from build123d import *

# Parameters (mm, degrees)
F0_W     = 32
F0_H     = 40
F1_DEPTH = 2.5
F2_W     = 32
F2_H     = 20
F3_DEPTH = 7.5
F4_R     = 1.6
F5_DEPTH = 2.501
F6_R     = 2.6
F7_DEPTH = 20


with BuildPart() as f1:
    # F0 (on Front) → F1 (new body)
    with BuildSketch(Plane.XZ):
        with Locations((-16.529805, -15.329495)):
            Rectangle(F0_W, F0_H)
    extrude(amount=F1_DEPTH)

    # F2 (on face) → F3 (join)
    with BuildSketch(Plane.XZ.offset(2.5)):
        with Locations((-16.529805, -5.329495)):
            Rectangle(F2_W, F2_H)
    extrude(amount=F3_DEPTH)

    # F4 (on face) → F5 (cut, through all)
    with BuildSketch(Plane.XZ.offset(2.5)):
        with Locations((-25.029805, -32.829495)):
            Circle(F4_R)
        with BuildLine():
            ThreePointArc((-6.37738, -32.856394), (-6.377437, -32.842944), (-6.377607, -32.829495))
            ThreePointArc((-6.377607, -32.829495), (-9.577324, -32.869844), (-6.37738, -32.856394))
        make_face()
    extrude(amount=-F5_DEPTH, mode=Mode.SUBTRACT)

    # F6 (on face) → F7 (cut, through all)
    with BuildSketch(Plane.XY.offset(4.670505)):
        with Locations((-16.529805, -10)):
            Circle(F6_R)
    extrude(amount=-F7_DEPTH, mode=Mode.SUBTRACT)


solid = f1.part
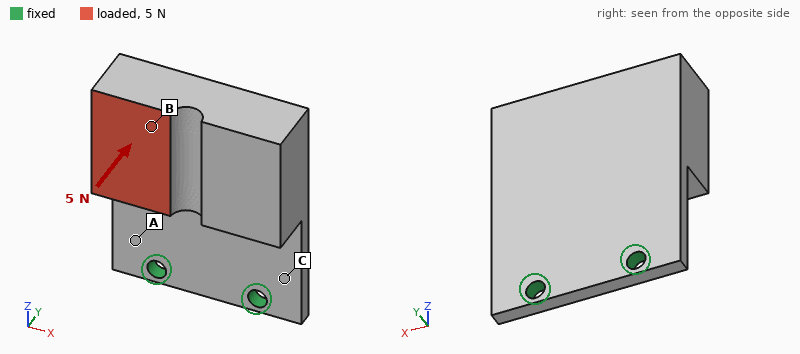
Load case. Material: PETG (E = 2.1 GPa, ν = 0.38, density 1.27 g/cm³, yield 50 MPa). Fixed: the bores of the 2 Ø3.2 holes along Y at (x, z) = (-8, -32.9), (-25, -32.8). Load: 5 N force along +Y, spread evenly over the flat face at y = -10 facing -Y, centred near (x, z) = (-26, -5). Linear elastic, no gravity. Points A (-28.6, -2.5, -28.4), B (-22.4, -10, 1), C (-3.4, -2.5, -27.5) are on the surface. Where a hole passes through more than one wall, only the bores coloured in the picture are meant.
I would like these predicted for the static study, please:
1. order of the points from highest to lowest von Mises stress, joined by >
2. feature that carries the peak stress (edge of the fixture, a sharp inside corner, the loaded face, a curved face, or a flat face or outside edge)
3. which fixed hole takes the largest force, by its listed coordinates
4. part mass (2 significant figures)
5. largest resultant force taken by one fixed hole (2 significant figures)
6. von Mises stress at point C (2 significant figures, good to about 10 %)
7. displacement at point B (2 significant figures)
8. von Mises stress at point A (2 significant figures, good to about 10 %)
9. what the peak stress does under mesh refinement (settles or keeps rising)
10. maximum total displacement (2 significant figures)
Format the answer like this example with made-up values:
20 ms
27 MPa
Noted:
A > C > B
edge of the fixture
(-25, -32.8)
9.8 g
4.8 N
2.7 MPa
0.52 mm
3.7 MPa
keeps rising
0.61 mm
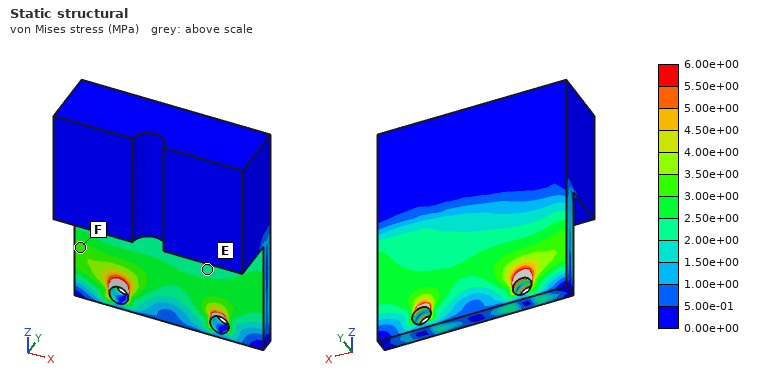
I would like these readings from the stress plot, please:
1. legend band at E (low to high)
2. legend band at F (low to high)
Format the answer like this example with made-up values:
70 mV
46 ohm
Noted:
2.00e+00 to 2.50e+00 MPa
3.00e+00 to 3.50e+00 MPa
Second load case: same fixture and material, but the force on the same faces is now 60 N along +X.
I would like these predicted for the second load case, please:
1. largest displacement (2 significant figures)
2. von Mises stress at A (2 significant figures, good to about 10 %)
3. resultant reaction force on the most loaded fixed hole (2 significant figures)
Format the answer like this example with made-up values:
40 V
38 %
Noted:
0.56 mm
5.5 MPa
93 N
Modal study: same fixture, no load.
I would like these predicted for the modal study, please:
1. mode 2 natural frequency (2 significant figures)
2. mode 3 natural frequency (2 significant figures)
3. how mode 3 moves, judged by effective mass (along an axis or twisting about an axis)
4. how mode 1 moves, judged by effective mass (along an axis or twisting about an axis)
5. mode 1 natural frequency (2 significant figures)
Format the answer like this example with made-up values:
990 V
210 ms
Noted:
710 Hz
1500 Hz
along X
along Y
200 Hz
